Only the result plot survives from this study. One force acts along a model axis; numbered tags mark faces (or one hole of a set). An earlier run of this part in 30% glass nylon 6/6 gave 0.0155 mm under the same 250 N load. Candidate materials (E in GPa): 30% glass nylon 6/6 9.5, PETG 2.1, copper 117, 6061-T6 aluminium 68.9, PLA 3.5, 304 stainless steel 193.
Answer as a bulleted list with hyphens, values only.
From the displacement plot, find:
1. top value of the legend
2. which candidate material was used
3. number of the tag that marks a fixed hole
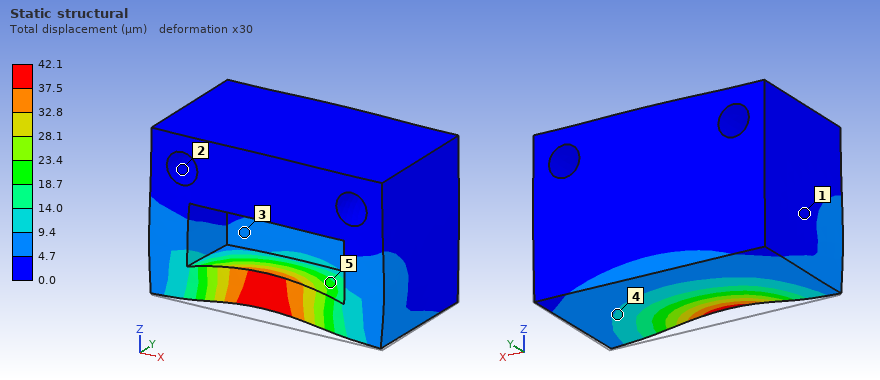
- 42.1 µm
- PLA
- 2
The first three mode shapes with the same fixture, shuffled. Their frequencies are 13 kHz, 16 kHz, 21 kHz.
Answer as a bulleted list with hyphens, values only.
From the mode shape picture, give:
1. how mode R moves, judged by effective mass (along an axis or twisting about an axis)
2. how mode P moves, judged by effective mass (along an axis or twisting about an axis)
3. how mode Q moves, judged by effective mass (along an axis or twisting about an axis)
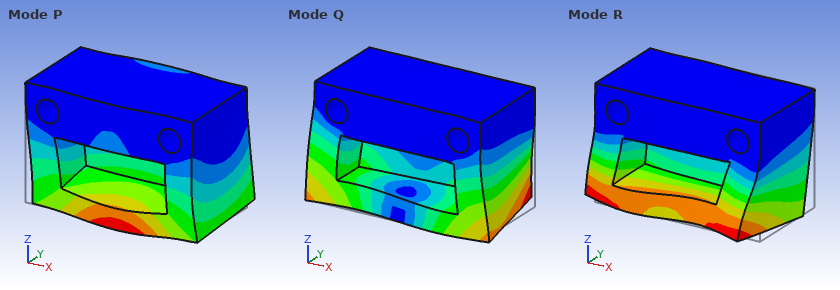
- along X
- along Y
- along X
